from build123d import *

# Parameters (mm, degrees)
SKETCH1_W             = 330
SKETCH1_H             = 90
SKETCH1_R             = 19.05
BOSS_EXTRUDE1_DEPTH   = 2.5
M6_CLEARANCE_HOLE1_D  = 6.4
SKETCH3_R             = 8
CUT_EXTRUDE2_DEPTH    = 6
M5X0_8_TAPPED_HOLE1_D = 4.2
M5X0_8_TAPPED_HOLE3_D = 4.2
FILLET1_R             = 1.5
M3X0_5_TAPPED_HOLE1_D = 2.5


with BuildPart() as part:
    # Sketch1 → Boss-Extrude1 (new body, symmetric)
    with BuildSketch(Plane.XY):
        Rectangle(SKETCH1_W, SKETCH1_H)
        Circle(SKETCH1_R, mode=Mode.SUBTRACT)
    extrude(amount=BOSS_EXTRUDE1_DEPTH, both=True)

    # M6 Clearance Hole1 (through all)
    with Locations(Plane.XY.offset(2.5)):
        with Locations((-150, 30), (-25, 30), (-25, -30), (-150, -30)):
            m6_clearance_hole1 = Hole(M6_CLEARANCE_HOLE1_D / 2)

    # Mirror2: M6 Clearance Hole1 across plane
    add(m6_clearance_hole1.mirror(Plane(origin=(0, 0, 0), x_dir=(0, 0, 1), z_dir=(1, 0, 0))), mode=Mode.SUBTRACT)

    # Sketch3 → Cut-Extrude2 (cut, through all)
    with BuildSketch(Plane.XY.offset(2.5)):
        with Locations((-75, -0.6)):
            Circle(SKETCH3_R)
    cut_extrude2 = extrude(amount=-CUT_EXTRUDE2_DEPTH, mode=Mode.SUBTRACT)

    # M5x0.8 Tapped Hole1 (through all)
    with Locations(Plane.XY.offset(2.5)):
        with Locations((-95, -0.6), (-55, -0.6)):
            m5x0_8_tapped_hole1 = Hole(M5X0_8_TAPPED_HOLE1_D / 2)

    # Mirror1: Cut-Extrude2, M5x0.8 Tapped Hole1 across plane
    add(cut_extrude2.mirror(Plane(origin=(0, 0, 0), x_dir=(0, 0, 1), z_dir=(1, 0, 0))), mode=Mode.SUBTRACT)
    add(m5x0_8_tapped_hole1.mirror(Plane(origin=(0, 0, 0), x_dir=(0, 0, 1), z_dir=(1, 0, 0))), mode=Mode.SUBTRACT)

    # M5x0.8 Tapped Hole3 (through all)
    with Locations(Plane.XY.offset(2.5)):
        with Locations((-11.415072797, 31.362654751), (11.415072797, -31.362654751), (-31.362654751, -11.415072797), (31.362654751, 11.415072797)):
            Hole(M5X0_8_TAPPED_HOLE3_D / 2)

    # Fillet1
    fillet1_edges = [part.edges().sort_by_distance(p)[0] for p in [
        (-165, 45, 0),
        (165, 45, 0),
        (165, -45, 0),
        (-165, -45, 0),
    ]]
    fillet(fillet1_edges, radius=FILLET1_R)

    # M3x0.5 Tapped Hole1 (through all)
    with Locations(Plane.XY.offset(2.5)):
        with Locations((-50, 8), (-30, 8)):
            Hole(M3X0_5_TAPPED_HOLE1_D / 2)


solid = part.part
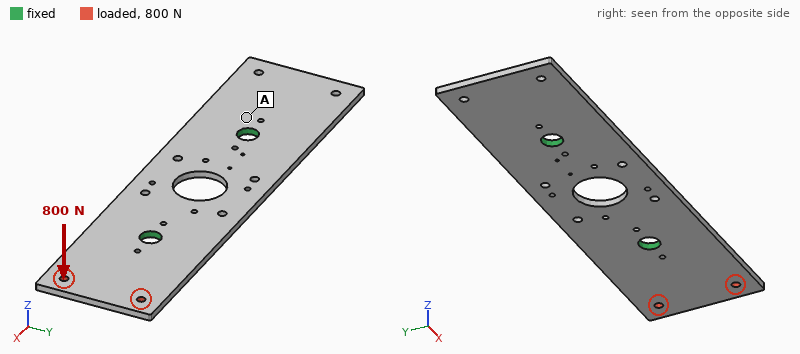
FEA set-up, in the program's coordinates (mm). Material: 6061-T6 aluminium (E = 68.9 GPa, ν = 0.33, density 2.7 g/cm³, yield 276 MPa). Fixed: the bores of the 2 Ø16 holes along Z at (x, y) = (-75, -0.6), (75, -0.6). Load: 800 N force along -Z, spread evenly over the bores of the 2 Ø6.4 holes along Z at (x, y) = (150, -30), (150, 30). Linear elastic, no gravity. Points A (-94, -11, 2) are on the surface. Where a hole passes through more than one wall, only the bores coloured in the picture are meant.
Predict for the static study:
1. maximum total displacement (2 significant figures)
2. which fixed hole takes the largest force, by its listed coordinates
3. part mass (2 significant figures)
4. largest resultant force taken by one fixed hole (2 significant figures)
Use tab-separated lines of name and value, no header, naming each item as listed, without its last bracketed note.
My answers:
maximum total displacement	2.1 mm
which fixed hole takes the largest force, by its listed coordinates	(75, -0.6)
part mass	380 g
largest resultant force taken by one fixed hole	830 N
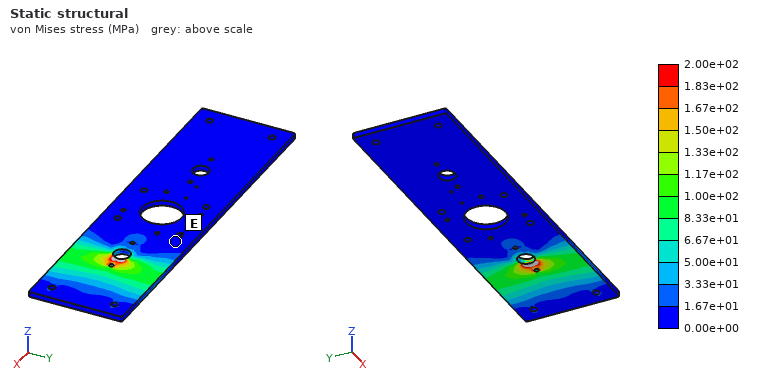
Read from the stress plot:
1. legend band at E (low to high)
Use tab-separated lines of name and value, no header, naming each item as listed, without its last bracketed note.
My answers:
legend band at E	0.00e+00 to 1.67e+01 MPa
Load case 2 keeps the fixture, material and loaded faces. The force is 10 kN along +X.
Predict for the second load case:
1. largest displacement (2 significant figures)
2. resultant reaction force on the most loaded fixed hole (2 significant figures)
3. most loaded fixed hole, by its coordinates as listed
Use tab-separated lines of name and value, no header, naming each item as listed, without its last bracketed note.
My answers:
largest displacement	41 µm
resultant reaction force on the most loaded fixed hole	8.9 kN
most loaded fixed hole, by its coordinates as listed	(75, -0.6)
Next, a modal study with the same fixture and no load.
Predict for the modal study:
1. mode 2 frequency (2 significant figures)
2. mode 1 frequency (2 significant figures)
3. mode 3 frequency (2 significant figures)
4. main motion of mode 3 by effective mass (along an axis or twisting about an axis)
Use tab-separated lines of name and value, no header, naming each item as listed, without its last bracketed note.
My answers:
mode 2 frequency	530 Hz
mode 1 frequency	530 Hz
mode 3 frequency	1000 Hz
main motion of mode 3 by effective mass	twisting about X
